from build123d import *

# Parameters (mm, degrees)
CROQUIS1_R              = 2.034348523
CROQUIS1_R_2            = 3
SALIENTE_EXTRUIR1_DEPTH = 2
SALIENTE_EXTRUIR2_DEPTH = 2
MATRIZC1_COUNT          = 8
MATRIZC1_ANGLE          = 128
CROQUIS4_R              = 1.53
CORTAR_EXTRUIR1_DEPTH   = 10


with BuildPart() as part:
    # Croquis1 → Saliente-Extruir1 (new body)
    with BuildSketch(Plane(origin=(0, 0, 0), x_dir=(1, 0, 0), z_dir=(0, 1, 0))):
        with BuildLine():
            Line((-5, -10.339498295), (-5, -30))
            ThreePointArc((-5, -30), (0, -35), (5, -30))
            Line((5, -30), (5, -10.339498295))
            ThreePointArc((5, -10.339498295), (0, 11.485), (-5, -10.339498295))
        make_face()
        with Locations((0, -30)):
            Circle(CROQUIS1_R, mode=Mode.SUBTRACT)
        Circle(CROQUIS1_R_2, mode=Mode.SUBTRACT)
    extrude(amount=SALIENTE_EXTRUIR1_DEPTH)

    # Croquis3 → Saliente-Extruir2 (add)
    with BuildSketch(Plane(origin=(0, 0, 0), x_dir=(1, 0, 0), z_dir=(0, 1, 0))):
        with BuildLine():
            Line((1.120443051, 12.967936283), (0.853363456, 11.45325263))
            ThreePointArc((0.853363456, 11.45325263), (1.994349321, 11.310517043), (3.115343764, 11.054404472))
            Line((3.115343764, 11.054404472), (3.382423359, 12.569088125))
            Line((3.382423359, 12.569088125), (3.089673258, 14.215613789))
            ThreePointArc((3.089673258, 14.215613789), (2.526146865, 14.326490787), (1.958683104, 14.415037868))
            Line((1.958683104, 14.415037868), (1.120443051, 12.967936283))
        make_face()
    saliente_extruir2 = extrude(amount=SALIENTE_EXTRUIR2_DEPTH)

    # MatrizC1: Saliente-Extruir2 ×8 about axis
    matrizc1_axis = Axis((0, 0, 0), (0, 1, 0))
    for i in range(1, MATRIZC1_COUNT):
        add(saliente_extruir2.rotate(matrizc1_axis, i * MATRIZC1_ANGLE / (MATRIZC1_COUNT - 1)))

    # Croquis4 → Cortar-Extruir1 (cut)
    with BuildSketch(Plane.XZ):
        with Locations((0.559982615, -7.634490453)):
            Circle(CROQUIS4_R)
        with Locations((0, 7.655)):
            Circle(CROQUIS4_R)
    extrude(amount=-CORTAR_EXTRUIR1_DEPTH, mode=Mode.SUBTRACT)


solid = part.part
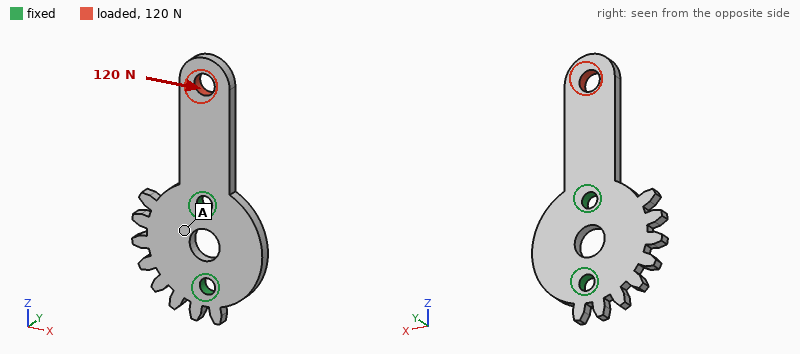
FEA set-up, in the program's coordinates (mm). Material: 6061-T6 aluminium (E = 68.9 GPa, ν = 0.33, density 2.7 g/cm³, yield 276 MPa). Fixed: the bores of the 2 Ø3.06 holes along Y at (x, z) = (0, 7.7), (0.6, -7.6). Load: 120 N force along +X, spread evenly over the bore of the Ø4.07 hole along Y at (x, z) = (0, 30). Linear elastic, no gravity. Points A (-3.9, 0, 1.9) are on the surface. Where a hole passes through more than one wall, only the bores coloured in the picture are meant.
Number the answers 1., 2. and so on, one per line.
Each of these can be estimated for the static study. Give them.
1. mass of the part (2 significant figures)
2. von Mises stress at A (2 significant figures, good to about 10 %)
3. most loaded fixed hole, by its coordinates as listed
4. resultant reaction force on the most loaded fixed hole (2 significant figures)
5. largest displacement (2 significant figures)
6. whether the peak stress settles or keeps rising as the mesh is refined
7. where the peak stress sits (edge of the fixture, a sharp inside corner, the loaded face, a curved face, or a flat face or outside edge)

1. 3.4 g
2. 13 MPa
3. (0, 7.7)
4. 220 N
5. 66 µm
6. keeps rising
7. a sharp inside corner
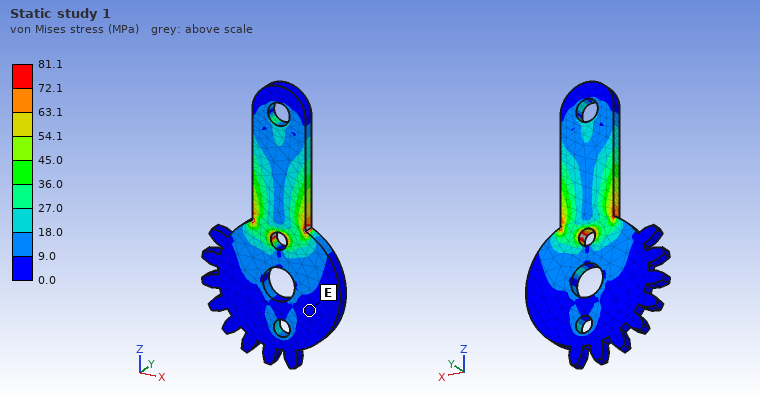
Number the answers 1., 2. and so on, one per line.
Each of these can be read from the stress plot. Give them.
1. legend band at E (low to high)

1. 0.0 to 9.0 MPa
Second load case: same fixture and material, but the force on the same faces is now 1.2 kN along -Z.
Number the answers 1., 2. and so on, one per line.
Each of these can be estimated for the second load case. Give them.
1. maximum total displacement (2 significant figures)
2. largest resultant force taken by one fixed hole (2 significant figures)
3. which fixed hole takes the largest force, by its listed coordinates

1. 26 µm
2. 1.1 kN
3. (0, 7.7)
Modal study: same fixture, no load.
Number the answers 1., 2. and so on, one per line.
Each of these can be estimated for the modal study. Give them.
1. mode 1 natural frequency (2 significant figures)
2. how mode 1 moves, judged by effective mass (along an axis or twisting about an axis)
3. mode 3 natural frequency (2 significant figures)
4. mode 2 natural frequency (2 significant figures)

1. 2700 Hz
2. along Y
3. 11 kHz
4. 11 kHz
